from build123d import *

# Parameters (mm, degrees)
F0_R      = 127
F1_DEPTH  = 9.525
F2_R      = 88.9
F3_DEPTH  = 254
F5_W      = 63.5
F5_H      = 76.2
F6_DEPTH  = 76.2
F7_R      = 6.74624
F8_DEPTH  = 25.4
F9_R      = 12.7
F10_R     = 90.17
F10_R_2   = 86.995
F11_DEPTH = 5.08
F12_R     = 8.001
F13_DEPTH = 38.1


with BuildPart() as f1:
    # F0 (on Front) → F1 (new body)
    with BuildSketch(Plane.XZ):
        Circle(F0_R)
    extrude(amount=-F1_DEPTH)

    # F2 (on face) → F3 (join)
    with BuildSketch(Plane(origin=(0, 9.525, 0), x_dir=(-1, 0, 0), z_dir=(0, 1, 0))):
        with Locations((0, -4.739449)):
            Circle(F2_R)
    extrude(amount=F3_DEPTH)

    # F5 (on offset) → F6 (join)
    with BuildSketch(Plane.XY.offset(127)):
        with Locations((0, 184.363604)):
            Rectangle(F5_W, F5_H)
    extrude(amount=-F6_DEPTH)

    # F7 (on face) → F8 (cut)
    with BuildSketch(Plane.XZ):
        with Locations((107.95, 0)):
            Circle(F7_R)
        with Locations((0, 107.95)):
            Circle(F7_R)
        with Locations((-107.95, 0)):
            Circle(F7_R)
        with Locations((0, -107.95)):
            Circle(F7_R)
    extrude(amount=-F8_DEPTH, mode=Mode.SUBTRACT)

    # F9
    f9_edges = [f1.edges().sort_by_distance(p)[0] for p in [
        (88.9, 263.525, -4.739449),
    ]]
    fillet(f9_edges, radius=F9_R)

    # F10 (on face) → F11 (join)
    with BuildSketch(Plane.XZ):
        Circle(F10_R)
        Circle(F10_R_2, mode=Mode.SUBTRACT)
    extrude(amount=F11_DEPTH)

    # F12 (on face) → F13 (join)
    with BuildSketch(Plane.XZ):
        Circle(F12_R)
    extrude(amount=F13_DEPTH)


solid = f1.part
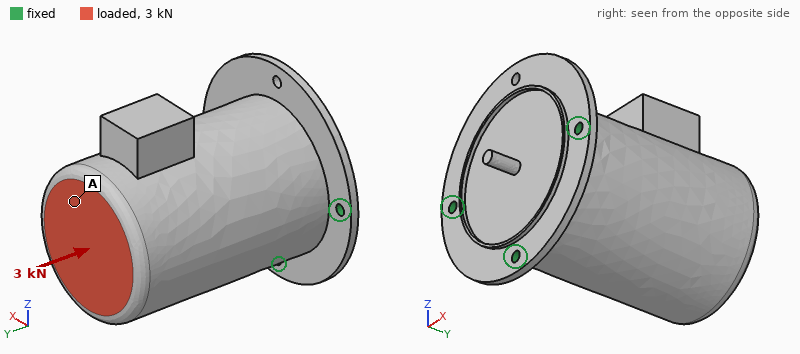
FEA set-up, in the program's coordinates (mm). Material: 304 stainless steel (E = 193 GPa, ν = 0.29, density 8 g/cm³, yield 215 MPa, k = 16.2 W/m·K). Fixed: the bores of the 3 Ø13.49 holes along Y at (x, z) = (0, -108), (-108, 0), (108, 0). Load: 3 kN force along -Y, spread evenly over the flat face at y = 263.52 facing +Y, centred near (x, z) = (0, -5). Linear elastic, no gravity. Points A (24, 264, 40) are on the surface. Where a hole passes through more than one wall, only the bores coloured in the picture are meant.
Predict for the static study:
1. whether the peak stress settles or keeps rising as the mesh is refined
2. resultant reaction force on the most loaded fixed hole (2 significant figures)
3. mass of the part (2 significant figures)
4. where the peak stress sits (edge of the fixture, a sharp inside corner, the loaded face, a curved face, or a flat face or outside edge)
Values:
keeps rising
1.5 kN
56 kg
edge of the fixture
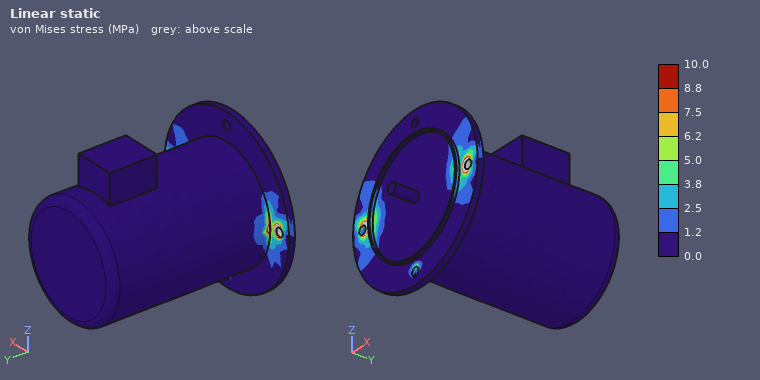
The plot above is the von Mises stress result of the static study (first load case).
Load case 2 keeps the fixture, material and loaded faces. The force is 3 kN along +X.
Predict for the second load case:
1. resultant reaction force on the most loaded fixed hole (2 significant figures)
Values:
4.3 kN
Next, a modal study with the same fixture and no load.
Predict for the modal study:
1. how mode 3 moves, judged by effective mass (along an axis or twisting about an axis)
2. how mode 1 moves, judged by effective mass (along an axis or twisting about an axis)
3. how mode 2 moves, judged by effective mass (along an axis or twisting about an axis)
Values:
along Y
along Z
along X
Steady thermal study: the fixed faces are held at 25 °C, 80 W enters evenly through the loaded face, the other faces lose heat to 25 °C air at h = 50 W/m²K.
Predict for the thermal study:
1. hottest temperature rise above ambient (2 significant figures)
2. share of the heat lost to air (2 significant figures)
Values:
27 K
97 %
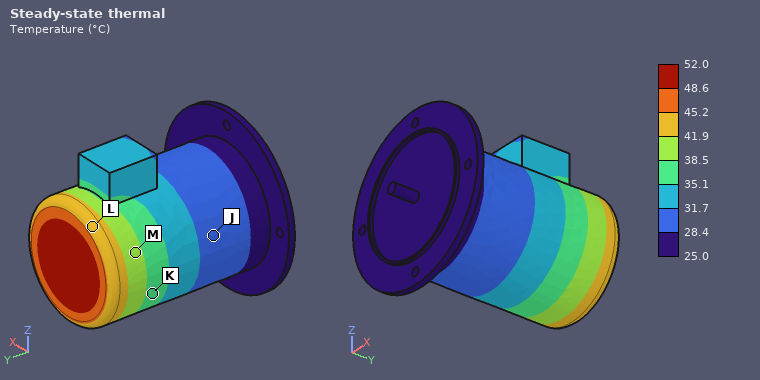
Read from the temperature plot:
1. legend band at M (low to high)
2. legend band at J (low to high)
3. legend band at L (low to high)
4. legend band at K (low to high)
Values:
38.5 to 41.9 °C
28.4 to 31.7 °C
41.9 to 45.2 °C
35.1 to 38.5 °C
